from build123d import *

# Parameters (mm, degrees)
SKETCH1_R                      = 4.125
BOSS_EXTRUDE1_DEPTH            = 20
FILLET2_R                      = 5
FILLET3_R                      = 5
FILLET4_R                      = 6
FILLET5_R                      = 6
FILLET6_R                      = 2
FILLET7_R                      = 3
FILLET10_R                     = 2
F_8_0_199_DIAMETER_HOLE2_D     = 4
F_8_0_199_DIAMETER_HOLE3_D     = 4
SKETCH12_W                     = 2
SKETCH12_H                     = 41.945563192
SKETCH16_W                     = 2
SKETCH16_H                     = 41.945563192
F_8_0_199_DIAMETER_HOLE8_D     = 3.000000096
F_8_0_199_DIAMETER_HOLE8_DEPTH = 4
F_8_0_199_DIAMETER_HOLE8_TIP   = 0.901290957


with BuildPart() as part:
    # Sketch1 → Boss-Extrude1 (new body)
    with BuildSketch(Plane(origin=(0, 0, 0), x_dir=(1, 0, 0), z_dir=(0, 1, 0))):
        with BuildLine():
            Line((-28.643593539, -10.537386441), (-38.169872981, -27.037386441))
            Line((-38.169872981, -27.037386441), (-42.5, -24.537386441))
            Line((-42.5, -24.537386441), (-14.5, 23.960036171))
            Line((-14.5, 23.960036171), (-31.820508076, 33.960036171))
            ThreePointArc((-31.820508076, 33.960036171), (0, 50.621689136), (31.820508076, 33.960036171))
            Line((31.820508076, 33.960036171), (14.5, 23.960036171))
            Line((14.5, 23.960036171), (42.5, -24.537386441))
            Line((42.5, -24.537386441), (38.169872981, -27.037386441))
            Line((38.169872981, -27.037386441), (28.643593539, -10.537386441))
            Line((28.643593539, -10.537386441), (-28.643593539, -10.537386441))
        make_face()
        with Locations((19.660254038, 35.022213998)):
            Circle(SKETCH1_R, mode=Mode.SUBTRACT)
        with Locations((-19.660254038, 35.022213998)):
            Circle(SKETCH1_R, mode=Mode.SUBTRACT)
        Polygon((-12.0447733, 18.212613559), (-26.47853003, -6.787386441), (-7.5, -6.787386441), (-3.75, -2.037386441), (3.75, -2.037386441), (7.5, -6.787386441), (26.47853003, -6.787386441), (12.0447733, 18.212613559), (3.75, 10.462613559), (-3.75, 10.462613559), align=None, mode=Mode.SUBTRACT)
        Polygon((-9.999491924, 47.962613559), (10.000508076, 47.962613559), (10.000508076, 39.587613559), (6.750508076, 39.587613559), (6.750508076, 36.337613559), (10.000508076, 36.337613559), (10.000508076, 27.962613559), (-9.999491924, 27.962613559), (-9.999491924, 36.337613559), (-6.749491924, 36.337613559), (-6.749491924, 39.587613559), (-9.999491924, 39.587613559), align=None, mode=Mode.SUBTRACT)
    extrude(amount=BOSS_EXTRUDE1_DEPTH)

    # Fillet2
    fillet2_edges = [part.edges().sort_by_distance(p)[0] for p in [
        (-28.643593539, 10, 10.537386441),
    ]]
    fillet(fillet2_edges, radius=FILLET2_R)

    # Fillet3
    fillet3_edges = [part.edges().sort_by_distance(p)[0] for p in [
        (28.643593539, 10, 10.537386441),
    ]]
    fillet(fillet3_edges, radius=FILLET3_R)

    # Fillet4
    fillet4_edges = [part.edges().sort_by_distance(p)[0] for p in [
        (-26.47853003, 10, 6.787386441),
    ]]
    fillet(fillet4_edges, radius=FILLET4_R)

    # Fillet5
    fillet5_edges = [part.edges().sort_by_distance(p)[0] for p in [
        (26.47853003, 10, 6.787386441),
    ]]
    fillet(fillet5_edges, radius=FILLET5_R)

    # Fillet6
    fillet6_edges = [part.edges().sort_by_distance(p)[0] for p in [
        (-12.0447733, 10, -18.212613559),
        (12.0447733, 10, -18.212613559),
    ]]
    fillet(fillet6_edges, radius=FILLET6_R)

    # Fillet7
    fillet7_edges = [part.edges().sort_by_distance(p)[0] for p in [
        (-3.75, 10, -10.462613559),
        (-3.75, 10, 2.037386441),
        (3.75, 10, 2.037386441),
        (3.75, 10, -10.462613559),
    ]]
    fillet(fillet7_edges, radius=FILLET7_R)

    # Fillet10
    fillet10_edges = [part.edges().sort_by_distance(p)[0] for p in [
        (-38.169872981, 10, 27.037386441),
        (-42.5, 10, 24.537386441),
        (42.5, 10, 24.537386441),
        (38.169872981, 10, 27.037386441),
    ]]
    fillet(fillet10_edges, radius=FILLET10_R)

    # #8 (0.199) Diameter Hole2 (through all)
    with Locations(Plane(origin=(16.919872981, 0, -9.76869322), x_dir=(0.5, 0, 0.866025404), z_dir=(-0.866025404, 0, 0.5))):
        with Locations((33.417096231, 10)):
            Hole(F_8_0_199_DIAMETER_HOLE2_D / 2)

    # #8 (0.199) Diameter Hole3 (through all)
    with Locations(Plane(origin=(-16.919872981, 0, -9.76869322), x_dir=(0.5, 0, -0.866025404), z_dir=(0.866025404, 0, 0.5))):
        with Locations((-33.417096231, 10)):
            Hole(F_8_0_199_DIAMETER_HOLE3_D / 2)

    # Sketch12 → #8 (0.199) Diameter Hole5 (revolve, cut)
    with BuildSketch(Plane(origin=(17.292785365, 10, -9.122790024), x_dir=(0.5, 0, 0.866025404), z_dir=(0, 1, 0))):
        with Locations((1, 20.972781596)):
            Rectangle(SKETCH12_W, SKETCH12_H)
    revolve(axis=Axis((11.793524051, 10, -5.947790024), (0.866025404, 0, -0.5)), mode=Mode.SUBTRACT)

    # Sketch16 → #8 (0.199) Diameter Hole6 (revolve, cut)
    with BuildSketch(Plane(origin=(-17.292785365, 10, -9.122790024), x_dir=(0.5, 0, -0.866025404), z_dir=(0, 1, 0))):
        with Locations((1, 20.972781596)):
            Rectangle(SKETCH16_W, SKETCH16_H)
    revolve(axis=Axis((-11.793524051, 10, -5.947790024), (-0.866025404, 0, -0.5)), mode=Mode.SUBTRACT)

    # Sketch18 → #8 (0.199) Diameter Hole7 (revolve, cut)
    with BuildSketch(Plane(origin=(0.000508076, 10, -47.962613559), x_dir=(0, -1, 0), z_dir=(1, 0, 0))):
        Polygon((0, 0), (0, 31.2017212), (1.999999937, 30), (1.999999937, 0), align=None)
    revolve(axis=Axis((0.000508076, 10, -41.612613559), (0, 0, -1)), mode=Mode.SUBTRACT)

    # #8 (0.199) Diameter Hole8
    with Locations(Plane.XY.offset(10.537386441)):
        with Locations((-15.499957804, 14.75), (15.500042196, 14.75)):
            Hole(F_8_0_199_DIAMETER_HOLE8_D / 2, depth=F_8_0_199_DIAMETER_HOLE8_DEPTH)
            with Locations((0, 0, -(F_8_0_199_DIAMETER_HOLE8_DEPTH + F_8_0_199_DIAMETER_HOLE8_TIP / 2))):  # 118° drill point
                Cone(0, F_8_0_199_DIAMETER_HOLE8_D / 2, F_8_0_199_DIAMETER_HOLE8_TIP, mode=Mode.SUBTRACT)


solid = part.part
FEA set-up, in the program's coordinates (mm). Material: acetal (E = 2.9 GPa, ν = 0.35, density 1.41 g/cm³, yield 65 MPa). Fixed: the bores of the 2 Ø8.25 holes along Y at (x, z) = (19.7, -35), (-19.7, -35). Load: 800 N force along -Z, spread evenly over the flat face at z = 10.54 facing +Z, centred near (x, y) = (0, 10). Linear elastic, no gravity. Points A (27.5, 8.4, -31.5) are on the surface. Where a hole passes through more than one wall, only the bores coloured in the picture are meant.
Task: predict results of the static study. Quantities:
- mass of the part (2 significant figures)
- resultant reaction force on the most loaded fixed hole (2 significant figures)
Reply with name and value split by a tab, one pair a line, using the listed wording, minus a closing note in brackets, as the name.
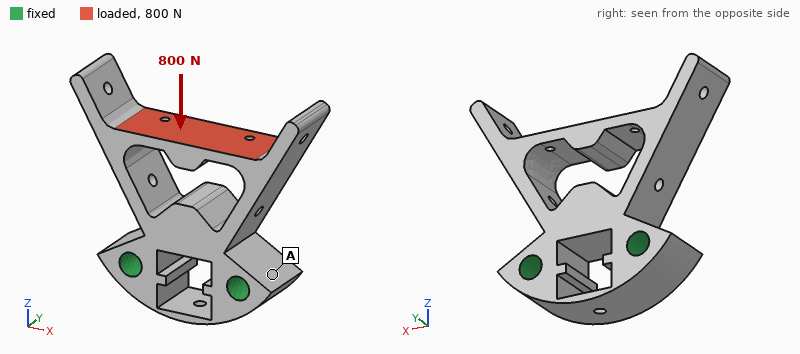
mass of the part	52 g
resultant reaction force on the most loaded fixed hole	400 N
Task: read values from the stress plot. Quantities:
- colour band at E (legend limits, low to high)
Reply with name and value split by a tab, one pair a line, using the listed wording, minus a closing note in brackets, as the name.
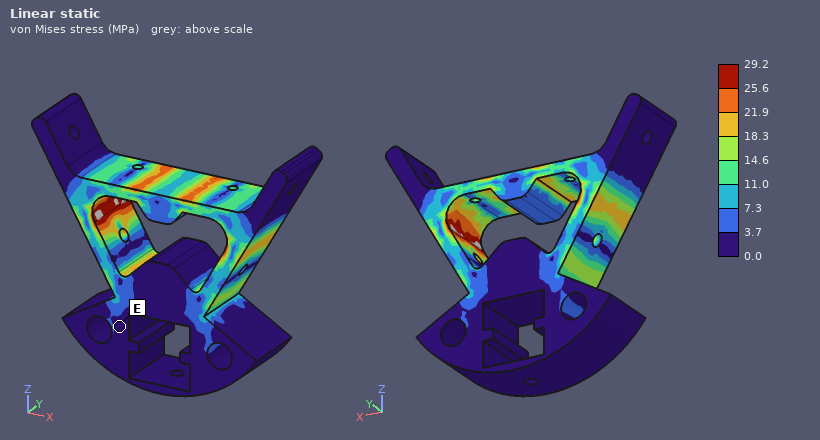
colour band at E	0.0 to 3.7 MPa
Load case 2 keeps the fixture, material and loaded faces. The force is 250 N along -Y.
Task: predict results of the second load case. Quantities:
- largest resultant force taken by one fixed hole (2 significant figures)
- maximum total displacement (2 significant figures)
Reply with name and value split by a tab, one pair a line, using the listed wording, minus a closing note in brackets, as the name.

largest resultant force taken by one fixed hole	130 N
maximum total displacement	0.70 mm
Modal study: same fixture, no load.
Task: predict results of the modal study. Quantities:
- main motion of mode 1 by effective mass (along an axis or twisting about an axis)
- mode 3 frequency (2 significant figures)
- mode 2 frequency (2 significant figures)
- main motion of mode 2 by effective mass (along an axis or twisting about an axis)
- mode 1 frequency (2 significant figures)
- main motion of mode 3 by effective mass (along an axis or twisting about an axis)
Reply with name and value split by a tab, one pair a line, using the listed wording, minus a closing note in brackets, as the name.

main motion of mode 1 by effective mass	along X
mode 3 frequency	1100 Hz
mode 2 frequency	860 Hz
main motion of mode 2 by effective mass	along Y
mode 1 frequency	460 Hz
main motion of mode 3 by effective mass	twisting about Z
